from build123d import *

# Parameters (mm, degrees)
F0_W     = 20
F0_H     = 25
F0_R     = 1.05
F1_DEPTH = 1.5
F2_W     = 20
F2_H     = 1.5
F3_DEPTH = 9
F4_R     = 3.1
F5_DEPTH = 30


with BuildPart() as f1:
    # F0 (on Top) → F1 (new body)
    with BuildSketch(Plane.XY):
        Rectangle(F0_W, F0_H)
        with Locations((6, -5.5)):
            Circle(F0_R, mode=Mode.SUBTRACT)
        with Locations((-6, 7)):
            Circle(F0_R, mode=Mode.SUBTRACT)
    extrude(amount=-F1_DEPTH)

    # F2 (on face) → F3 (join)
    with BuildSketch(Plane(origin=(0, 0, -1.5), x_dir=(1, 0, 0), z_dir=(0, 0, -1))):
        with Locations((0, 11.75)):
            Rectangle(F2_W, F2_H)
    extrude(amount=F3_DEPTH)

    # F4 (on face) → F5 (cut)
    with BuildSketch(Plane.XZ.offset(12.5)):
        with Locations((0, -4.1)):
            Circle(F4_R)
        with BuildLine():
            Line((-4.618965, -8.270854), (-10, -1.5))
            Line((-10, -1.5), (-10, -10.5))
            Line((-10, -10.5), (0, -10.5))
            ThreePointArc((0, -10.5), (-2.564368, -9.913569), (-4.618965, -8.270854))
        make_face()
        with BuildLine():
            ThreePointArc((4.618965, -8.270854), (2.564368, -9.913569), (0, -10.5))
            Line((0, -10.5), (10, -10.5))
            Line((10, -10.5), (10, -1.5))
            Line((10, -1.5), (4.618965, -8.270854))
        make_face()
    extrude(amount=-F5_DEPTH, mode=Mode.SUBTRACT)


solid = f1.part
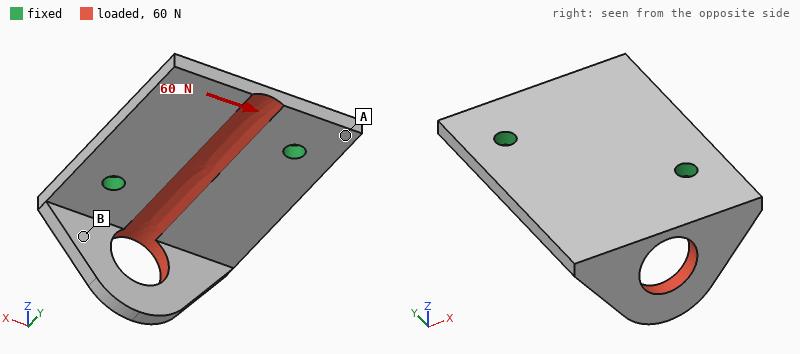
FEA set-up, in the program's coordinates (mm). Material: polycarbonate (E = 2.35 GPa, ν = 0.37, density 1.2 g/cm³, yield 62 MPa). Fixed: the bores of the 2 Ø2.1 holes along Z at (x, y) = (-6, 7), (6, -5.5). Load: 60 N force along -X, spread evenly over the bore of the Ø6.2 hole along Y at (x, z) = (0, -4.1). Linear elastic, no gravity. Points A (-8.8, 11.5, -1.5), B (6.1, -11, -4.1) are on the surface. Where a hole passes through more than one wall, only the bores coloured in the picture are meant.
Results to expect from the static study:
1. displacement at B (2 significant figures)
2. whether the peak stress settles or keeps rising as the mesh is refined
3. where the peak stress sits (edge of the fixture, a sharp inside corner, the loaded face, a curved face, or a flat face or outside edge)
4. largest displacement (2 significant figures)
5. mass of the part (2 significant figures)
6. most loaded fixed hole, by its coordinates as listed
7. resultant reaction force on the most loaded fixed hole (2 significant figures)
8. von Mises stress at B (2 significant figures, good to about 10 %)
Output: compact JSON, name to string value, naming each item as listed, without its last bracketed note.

{"displacement at B": "0.083 mm", "whether the peak stress settles or keeps rising as the mesh is refined": "keeps rising", "where the peak stress sits": "edge of the fixture", "largest displacement": "0.33 mm", "mass of the part": "1.0 g", "most loaded fixed hole, by its coordinates as listed": "(6, -5.5)", "resultant reaction force on the most loaded fixed hole": "39 N", "von Mises stress at B": "4.1 MPa"}
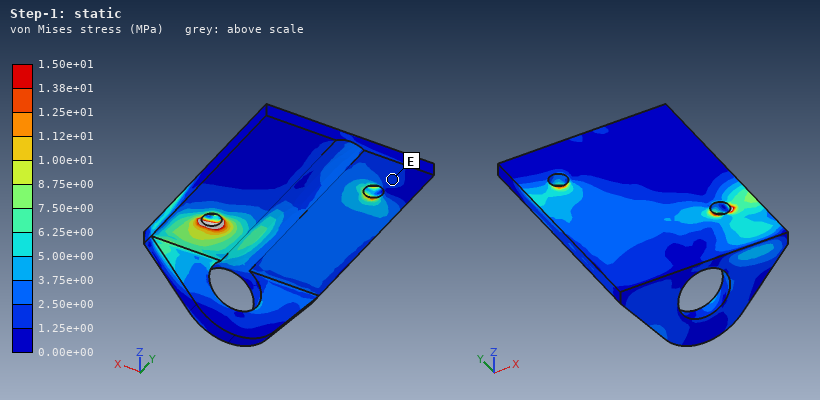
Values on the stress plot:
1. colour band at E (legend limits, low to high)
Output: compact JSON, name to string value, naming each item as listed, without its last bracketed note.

{"colour band at E": "1.25e+00 to 2.50e+00 MPa"}
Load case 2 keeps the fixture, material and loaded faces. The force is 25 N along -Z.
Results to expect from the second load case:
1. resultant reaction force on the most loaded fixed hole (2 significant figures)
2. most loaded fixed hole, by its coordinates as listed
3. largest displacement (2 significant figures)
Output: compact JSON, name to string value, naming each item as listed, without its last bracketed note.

{"resultant reaction force on the most loaded fixed hole": "16 N", "most loaded fixed hole, by its coordinates as listed": "(6, -5.5)", "largest displacement": "0.39 mm"}
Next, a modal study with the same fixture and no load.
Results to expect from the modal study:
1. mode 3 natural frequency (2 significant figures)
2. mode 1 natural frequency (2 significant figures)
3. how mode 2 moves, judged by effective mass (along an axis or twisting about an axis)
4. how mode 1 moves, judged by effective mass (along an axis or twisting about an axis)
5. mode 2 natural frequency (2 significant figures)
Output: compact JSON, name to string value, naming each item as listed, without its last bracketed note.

{"mode 3 natural frequency": "2700 Hz", "mode 1 natural frequency": "1500 Hz", "how mode 2 moves, judged by effective mass": "along Z", "how mode 1 moves, judged by effective mass": "along Z", "mode 2 natural frequency": "2200 Hz"}
